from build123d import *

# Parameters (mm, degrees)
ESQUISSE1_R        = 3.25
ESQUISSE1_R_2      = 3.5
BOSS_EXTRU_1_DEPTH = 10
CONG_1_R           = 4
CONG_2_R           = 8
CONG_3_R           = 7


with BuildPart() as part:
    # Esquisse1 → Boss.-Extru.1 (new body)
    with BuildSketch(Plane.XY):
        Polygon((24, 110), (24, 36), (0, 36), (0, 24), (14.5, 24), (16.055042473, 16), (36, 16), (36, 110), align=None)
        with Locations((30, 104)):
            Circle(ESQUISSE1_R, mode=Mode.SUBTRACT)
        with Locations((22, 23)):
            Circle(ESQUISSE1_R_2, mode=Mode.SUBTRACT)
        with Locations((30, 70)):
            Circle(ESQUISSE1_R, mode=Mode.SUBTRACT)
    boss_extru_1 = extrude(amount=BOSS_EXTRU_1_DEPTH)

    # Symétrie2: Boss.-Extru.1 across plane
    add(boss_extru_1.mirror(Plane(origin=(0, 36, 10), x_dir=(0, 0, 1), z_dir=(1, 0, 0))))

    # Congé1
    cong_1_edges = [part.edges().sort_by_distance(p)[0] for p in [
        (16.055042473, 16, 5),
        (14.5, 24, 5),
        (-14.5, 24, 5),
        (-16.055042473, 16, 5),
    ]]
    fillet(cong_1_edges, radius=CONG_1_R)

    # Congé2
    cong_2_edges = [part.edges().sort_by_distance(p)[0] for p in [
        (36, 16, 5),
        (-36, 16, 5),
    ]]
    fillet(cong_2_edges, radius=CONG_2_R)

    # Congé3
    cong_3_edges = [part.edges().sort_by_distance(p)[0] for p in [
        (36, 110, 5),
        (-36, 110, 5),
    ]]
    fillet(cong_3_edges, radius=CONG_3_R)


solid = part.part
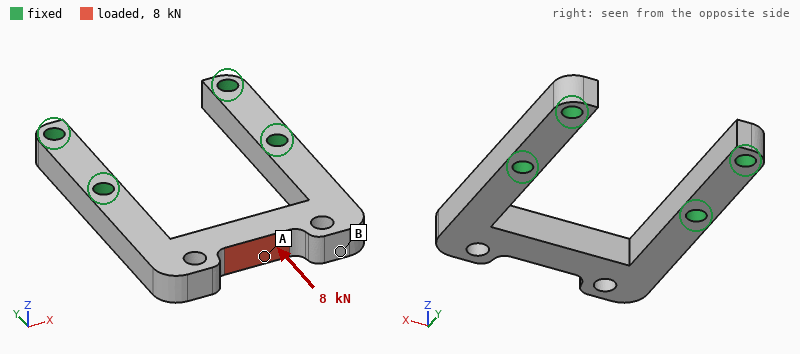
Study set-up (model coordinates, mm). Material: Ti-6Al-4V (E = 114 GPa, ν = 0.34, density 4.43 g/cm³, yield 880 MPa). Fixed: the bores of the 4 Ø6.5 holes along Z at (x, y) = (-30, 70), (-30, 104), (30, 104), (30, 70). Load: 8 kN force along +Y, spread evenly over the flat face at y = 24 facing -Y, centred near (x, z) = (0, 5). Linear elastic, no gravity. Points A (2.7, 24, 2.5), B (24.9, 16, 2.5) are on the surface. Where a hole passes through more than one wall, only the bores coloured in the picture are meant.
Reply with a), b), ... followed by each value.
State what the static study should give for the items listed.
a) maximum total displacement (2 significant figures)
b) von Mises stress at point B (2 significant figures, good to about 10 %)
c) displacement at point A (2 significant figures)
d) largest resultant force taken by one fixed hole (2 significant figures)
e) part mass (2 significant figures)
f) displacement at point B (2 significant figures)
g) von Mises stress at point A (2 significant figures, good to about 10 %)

a) 0.10 mm
b) 29 MPa
c) 0.099 mm
d) 4.3 kN
e) 120 g
f) 0.054 mm
g) 210 MPa
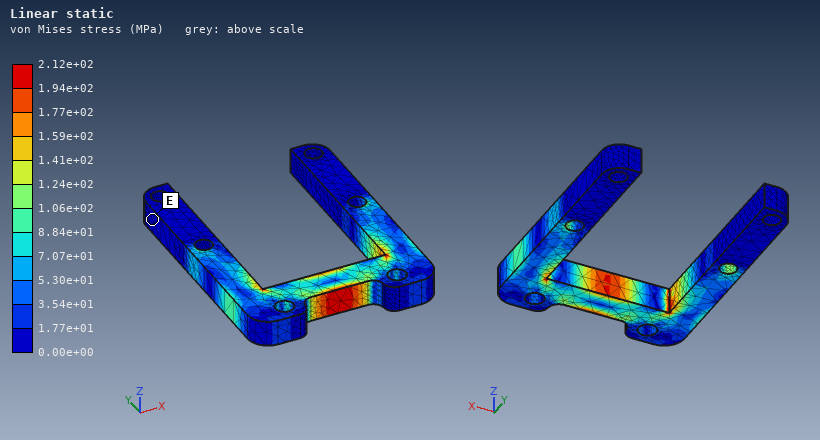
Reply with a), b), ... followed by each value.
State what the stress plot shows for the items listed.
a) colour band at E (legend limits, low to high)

a) 0.00e+00 to 1.77e+01 MPa
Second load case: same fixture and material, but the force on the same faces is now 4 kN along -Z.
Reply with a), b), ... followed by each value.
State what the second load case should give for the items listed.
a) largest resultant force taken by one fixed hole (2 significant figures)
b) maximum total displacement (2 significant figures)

a) 2.1 kN
b) 0.72 mm
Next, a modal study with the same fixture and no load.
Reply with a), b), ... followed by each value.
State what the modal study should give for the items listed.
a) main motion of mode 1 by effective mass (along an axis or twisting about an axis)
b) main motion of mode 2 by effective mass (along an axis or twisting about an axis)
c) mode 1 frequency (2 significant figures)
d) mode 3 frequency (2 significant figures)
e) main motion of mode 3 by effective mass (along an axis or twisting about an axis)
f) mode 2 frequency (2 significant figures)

a) along Z
b) twisting about Y
c) 2100 Hz
d) 4100 Hz
e) along X
f) 3900 Hz
